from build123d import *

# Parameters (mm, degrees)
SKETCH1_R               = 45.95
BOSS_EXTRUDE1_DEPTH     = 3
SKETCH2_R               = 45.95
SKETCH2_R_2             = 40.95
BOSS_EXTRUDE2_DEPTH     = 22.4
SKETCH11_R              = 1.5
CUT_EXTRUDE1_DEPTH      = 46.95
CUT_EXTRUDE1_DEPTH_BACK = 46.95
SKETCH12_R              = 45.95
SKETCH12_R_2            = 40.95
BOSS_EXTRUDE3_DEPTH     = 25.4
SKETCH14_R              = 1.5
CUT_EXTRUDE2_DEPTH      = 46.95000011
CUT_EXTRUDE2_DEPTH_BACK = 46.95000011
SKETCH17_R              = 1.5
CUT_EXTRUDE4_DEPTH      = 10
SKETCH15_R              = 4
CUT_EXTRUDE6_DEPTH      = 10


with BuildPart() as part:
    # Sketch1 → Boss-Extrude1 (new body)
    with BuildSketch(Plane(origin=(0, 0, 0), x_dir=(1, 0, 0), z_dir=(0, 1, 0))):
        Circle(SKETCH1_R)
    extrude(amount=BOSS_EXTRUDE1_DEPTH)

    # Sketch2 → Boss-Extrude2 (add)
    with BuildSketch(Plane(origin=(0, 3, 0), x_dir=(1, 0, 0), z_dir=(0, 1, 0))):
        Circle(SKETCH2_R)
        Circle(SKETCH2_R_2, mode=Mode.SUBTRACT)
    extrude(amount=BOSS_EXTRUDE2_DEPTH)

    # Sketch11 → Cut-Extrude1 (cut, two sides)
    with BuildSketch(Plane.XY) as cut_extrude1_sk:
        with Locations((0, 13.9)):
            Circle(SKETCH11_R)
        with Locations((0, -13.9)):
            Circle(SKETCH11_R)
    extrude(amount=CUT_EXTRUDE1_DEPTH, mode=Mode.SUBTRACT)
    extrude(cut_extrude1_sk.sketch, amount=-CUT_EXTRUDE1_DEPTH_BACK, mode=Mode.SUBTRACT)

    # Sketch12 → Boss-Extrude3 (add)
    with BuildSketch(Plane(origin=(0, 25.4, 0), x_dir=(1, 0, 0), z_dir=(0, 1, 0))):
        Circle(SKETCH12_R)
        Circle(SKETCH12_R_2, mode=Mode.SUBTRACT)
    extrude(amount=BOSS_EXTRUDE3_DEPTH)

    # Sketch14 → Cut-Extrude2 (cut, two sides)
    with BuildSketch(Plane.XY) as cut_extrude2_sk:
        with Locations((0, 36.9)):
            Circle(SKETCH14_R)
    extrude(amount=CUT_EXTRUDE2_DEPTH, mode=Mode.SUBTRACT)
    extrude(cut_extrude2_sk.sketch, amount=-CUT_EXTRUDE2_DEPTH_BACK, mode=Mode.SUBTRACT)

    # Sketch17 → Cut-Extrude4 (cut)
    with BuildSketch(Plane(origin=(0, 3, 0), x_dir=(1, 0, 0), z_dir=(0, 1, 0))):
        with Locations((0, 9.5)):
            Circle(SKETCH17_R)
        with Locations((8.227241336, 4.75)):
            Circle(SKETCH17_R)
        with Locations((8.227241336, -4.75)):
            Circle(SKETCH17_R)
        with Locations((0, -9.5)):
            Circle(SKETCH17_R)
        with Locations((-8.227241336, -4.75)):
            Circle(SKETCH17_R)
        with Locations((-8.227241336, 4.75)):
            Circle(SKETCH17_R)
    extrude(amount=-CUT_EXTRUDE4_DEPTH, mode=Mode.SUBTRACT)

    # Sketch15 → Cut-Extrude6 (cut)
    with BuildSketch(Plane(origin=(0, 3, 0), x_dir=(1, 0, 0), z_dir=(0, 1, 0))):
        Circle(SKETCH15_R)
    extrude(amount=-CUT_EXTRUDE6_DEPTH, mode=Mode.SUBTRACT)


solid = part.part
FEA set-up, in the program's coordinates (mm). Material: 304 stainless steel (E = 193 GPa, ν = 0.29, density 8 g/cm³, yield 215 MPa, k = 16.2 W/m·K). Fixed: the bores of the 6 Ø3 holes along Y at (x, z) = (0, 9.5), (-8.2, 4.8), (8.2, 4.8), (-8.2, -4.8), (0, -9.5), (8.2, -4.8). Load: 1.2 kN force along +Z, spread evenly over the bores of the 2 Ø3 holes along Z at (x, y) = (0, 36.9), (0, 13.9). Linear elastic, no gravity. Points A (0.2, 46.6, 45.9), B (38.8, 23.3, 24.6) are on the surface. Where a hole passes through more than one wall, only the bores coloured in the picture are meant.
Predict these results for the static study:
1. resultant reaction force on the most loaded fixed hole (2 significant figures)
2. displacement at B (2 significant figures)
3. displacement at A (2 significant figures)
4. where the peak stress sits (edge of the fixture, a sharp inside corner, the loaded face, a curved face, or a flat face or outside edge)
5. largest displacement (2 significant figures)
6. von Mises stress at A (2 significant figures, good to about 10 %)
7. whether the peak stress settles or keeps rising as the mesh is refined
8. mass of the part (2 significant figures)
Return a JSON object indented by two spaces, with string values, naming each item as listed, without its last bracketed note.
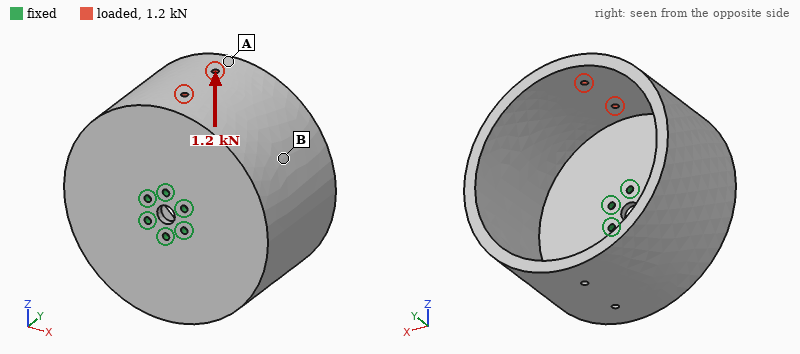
{
  "resultant reaction force on the most loaded fixed hole": "550 N",
  "displacement at B": "0.099 mm",
  "displacement at A": "0.22 mm",
  "where the peak stress sits": "edge of the fixture",
  "largest displacement": "0.23 mm",
  "von Mises stress at A": "37 MPa",
  "whether the peak stress settles or keeps rising as the mesh is refined": "keeps rising",
  "mass of the part": "680 g"
}
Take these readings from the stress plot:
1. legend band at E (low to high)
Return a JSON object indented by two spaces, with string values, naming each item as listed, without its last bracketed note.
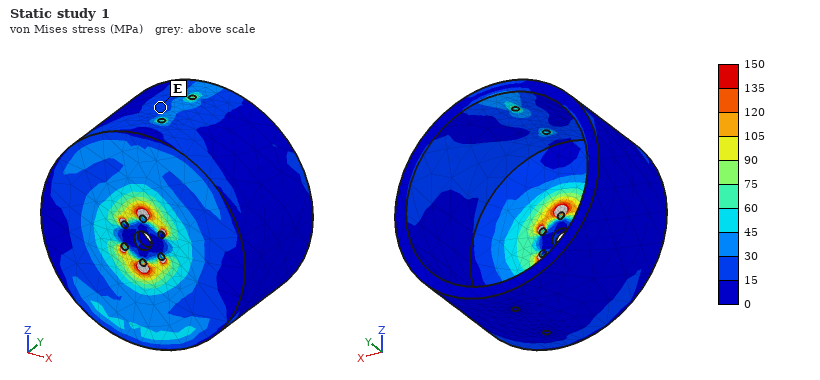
{
  "legend band at E": "15 to 30 MPa"
}
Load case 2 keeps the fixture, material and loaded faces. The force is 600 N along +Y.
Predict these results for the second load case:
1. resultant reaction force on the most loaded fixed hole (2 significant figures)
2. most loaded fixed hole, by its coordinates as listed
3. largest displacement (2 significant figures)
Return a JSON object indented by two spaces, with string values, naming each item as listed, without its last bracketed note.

{
  "resultant reaction force on the most loaded fixed hole": "580 N",
  "most loaded fixed hole, by its coordinates as listed": "(0, 9.5)",
  "largest displacement": "0.20 mm"
}
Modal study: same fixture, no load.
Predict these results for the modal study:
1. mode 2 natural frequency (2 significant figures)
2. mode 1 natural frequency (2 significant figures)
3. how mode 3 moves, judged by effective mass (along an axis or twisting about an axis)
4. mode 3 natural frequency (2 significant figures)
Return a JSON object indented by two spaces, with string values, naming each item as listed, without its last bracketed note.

{
  "mode 2 natural frequency": "500 Hz",
  "mode 1 natural frequency": "490 Hz",
  "how mode 3 moves, judged by effective mass": "along Y",
  "mode 3 natural frequency": "1000 Hz"
}
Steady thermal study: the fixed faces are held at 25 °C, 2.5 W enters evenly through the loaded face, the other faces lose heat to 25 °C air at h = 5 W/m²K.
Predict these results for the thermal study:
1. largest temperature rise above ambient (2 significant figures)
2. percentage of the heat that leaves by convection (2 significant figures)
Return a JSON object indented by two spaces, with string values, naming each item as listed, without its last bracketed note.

{
  "largest temperature rise above ambient": "20 K",
  "percentage of the heat that leaves by convection": "51 %"
}
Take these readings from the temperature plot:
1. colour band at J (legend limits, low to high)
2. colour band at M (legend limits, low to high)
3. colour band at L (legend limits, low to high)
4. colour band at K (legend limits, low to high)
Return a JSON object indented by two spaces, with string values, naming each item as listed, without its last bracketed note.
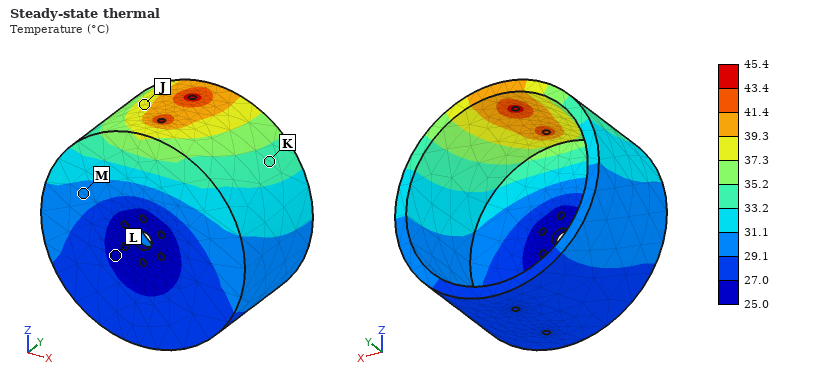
{
  "colour band at J": "37.3 to 39.3 °C",
  "colour band at M": "29.1 to 31.1 °C",
  "colour band at L": "25.0 to 27.0 °C",
  "colour band at K": "33.2 to 35.2 °C"
}
